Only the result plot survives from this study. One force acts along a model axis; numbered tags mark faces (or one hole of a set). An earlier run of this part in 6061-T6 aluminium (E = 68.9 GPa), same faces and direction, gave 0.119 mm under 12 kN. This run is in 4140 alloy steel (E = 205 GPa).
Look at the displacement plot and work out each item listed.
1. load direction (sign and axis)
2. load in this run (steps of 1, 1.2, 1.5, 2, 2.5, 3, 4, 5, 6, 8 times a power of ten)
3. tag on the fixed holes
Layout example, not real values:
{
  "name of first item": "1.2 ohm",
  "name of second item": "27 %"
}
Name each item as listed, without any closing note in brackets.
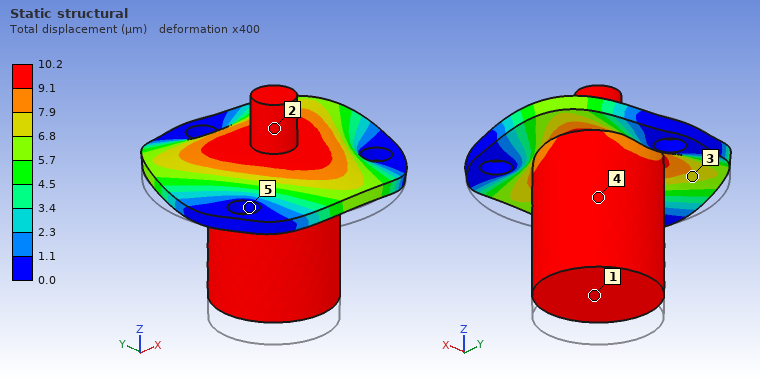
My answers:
{
  "load direction": "+Z",
  "load in this run": "3 kN",
  "tag on the fixed holes": "5"
}
